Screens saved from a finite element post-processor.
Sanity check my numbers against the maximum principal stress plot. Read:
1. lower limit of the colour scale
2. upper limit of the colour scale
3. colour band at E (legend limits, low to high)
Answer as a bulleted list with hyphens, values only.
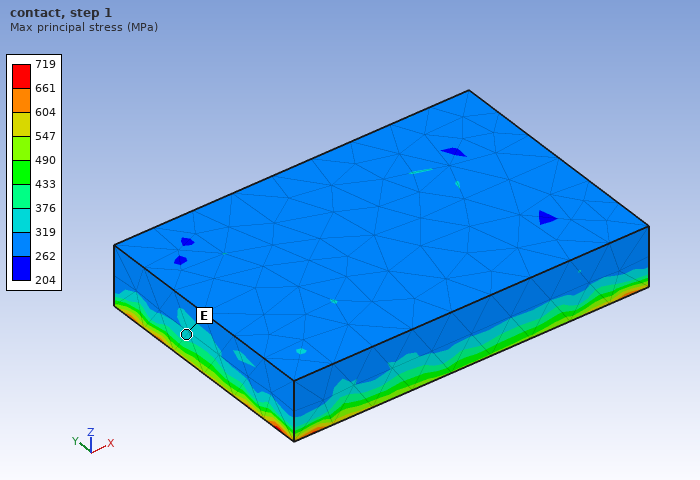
- 204 MPa
- 719 MPa
- 319 to 376 MPa
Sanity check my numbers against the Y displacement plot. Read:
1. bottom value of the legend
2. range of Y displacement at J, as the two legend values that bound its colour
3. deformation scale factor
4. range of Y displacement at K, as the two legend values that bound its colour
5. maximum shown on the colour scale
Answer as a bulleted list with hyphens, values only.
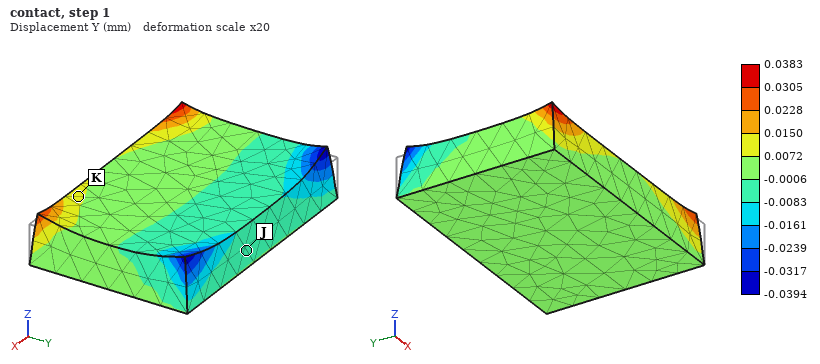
- -0.0394 mm
- -0.0083 to -0.0006 mm
- 20
- 0.0072 to 0.0150 mm
- 0.0383 mm
